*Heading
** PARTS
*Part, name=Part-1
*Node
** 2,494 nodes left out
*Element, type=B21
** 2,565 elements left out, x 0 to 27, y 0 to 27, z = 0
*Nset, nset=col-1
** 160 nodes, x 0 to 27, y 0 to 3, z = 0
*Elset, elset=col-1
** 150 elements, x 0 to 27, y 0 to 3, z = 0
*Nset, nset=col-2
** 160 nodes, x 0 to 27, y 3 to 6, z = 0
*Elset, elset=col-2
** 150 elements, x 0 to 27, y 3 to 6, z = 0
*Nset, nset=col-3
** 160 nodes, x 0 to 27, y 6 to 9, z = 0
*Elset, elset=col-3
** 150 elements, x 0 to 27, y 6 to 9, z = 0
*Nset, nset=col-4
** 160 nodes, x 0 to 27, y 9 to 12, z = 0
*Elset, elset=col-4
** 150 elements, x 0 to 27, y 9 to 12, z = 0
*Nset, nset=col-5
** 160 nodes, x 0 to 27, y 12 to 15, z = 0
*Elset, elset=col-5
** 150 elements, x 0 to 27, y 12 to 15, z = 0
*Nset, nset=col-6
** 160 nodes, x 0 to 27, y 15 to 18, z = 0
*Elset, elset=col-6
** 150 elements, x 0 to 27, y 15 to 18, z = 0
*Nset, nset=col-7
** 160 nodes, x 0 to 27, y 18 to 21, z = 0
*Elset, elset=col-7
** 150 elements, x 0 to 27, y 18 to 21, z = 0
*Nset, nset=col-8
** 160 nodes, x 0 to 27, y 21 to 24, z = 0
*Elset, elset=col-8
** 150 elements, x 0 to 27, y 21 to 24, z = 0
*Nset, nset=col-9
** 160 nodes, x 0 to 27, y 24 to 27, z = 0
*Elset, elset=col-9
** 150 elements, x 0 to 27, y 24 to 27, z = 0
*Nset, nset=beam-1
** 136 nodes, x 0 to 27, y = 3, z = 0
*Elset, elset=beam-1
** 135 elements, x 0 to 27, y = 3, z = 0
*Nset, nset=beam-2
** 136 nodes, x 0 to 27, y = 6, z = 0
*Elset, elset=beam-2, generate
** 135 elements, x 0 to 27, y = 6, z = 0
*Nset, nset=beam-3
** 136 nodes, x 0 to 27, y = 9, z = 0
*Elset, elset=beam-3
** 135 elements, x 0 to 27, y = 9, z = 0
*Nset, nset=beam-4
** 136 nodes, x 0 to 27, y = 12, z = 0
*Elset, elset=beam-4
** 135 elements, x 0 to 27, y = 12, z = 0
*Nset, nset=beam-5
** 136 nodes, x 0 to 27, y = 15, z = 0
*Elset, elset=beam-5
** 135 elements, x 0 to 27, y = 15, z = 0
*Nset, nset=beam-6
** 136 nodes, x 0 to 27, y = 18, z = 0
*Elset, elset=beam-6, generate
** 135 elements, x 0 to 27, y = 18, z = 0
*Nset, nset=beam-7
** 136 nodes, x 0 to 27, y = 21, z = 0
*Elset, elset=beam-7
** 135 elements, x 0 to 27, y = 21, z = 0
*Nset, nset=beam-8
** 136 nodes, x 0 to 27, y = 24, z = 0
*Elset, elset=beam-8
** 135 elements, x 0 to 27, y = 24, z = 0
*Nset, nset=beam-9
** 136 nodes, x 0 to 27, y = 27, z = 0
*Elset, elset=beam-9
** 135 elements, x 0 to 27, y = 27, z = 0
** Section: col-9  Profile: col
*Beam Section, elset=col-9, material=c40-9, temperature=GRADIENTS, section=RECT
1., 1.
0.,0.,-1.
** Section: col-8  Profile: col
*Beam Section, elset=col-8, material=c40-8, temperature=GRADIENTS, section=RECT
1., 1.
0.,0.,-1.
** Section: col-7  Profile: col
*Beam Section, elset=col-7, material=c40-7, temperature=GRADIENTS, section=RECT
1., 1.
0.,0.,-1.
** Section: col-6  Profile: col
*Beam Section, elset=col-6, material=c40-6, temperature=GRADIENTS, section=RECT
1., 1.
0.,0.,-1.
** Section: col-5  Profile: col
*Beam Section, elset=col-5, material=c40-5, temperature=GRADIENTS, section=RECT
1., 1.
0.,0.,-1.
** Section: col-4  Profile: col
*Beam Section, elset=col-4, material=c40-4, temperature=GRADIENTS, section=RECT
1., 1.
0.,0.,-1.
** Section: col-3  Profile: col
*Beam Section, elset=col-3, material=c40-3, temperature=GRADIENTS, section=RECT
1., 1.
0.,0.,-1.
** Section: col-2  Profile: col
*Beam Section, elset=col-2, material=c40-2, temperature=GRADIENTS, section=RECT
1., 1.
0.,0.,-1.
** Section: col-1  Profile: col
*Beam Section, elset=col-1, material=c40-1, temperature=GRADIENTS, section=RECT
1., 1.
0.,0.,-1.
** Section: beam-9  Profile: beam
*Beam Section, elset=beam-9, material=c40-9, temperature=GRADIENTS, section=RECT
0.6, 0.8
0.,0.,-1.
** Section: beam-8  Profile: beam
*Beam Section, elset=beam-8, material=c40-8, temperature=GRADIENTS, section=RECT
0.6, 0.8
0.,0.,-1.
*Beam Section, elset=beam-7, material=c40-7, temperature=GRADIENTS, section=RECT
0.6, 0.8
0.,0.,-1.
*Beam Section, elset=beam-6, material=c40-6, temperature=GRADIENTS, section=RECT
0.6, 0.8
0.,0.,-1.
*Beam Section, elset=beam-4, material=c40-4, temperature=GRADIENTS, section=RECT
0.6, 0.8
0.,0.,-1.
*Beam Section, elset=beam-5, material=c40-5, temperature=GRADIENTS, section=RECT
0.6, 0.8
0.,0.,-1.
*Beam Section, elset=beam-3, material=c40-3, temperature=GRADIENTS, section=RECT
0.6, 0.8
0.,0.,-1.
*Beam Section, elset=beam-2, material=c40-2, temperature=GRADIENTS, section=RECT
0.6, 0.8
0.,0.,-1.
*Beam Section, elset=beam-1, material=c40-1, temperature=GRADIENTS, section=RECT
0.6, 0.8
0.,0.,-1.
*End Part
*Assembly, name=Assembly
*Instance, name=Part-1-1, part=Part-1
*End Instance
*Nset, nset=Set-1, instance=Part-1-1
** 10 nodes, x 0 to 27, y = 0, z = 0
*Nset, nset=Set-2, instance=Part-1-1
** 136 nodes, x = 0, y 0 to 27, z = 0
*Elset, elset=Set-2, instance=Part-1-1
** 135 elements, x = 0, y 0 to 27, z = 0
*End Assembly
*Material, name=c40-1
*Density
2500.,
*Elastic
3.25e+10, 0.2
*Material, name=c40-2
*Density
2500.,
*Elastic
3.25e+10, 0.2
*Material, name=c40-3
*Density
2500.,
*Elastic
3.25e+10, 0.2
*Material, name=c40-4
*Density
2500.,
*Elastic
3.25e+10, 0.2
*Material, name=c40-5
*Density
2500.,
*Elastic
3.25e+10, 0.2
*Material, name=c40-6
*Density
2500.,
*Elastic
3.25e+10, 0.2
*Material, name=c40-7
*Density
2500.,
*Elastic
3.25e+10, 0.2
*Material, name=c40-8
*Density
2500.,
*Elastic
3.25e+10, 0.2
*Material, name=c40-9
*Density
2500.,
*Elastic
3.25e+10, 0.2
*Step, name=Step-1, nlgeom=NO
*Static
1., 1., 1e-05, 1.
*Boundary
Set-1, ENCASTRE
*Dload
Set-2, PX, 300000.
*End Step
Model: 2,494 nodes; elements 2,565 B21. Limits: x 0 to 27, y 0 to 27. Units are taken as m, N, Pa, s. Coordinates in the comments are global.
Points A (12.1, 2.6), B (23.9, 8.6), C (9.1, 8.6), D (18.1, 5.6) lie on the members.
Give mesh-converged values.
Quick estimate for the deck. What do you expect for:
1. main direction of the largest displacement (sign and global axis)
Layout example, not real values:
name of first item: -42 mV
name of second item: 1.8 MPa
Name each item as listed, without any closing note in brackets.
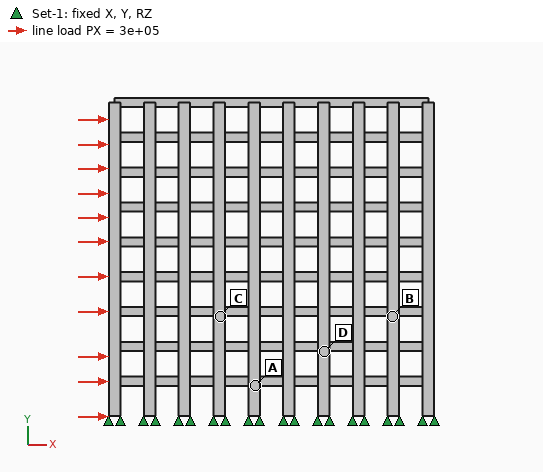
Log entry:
main direction of the largest displacement: +X
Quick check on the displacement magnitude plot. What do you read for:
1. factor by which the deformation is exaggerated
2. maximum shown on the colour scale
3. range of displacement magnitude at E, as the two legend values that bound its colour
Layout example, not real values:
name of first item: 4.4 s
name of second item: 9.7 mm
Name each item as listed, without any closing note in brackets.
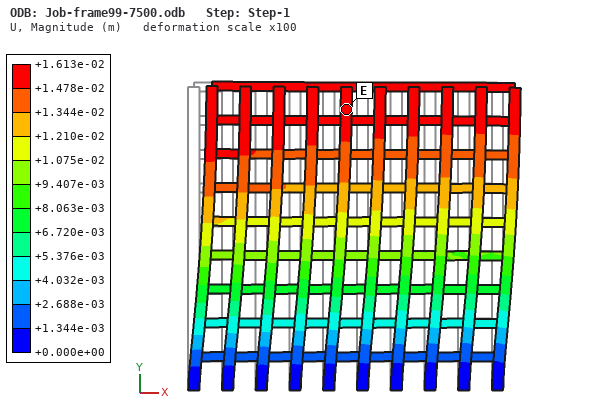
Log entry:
factor by which the deformation is exaggerated: 100
maximum shown on the colour scale: +1.613e-02 m
range of displacement magnitude at E, as the two legend values that bound its colour: +1.478e-02 to +1.613e-02 m
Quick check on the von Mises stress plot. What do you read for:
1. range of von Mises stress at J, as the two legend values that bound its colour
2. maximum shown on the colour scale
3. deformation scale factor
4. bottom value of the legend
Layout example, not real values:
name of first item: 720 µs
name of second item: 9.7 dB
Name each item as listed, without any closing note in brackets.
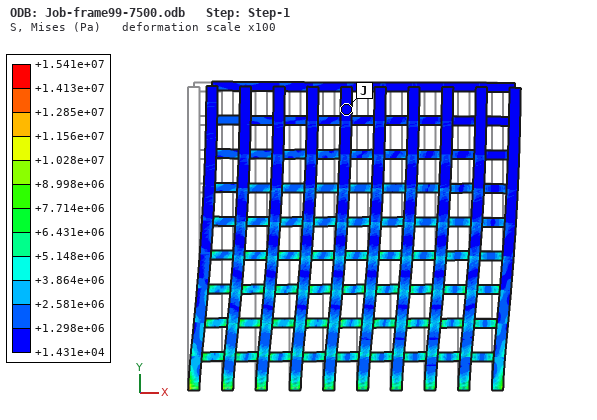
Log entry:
range of von Mises stress at J, as the two legend values that bound its colour: +1.431e+04 to +1.298e+06 Pa
maximum shown on the colour scale: +1.541e+07 Pa
deformation scale factor: 100
bottom value of the legend: +1.431e+04 Pa
